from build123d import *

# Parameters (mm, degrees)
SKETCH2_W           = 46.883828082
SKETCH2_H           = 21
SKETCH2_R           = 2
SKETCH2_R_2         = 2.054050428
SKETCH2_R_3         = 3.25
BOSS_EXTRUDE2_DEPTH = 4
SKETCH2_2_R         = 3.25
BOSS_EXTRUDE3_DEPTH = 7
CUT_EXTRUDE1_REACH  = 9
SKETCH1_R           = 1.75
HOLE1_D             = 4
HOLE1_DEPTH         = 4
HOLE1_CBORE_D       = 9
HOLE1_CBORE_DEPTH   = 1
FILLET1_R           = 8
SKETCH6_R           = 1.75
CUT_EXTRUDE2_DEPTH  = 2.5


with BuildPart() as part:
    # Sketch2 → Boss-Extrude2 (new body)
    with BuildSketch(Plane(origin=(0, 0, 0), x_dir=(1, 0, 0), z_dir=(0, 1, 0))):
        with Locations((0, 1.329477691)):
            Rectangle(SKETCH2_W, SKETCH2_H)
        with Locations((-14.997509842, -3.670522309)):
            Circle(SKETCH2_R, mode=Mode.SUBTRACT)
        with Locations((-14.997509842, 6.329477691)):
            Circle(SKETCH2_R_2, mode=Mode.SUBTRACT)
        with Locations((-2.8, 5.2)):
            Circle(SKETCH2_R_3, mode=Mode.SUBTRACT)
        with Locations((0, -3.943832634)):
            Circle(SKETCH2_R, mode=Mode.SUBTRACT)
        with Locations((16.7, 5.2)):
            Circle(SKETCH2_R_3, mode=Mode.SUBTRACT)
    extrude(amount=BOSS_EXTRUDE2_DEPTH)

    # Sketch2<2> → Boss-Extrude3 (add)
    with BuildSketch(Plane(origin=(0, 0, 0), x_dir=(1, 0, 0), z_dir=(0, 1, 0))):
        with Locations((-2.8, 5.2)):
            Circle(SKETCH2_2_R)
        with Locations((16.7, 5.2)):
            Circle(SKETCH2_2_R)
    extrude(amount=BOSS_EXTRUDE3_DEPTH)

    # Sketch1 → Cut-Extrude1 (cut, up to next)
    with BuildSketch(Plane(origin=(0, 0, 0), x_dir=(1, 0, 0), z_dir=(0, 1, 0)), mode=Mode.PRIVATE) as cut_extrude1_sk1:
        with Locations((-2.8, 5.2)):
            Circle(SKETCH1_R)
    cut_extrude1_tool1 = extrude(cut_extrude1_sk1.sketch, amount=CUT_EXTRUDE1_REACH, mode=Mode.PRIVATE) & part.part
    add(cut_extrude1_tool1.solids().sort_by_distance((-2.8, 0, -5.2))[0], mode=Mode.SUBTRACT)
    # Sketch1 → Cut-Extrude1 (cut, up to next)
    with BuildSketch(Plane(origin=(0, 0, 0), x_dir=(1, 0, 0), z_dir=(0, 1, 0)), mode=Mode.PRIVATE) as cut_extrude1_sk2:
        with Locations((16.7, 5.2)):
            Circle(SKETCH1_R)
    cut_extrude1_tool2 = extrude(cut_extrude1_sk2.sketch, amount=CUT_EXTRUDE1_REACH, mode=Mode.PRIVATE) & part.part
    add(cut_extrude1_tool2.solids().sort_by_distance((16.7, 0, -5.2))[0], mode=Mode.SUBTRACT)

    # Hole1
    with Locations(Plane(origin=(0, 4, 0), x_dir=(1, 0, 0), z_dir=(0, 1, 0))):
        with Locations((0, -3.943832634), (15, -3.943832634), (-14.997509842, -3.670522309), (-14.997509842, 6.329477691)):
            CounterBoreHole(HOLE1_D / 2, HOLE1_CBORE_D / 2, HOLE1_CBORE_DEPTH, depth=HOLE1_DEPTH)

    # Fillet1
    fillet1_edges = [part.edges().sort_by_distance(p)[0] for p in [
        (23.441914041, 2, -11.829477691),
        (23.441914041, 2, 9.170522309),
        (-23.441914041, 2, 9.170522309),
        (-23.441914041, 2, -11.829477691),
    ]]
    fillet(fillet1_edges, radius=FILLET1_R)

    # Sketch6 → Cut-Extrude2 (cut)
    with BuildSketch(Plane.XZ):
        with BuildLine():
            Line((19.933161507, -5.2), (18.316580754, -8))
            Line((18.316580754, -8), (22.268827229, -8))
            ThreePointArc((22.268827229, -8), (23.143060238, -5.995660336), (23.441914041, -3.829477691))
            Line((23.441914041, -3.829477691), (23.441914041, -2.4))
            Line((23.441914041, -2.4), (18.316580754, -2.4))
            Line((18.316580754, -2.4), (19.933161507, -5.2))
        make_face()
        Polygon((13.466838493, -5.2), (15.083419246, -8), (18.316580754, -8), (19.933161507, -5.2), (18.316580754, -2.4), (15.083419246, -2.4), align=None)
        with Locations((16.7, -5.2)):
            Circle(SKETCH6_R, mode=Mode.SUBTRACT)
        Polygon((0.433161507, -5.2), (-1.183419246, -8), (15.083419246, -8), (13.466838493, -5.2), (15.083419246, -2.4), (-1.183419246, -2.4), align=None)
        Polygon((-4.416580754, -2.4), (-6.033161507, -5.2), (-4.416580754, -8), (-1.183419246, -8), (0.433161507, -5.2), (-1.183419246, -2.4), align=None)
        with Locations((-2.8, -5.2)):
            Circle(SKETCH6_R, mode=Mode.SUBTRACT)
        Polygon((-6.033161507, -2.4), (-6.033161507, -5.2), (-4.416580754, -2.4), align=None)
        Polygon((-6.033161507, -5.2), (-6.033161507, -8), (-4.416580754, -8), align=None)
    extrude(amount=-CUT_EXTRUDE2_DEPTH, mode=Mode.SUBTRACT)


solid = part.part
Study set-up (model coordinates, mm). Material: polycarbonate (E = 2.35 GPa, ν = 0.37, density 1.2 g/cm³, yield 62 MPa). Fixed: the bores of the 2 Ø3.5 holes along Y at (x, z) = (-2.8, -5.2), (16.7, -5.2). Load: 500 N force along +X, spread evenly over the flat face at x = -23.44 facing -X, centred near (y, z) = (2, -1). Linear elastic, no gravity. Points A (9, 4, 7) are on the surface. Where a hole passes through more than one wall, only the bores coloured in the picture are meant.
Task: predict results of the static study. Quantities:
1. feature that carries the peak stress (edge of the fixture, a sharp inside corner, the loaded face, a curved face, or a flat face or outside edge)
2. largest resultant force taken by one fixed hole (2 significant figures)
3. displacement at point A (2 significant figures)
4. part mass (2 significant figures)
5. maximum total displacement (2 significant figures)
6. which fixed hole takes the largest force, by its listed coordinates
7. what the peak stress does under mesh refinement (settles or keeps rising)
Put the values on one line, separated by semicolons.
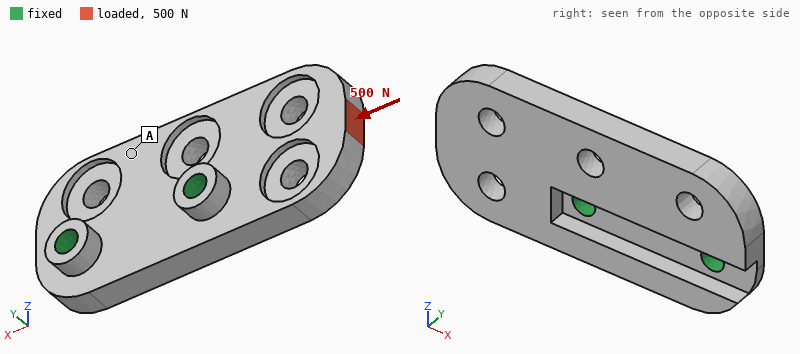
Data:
edge of the fixture; 360 N; 0.062 mm; 3.6 g; 0.22 mm; (-2.8, -5.2); keeps rising
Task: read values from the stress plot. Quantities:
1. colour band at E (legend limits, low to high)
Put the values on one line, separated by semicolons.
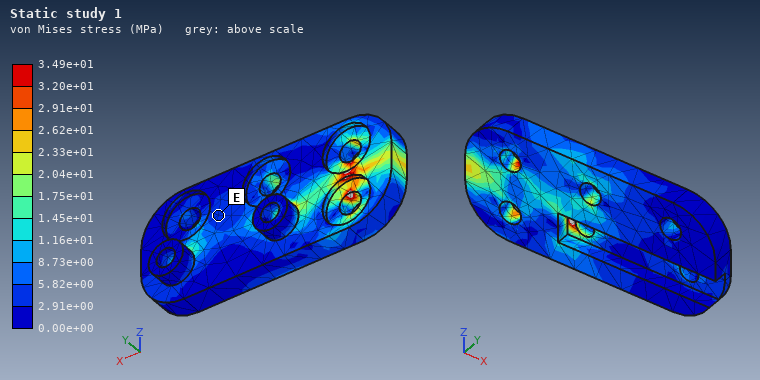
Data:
2.91e+00 to 5.82e+00 MPa
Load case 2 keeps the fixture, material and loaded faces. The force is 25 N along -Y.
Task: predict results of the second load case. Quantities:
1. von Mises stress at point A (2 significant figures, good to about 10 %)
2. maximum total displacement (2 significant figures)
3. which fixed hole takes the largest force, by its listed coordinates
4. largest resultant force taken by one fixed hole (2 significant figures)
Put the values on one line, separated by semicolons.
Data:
1.2 MPa; 0.59 mm; (-2.8, -5.2); 54 N
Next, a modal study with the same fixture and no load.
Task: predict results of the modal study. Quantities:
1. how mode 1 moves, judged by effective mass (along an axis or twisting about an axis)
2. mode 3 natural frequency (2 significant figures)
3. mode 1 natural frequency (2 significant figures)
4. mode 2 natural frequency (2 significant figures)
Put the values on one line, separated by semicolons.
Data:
along Y; 3500 Hz; 1700 Hz; 2200 Hz
